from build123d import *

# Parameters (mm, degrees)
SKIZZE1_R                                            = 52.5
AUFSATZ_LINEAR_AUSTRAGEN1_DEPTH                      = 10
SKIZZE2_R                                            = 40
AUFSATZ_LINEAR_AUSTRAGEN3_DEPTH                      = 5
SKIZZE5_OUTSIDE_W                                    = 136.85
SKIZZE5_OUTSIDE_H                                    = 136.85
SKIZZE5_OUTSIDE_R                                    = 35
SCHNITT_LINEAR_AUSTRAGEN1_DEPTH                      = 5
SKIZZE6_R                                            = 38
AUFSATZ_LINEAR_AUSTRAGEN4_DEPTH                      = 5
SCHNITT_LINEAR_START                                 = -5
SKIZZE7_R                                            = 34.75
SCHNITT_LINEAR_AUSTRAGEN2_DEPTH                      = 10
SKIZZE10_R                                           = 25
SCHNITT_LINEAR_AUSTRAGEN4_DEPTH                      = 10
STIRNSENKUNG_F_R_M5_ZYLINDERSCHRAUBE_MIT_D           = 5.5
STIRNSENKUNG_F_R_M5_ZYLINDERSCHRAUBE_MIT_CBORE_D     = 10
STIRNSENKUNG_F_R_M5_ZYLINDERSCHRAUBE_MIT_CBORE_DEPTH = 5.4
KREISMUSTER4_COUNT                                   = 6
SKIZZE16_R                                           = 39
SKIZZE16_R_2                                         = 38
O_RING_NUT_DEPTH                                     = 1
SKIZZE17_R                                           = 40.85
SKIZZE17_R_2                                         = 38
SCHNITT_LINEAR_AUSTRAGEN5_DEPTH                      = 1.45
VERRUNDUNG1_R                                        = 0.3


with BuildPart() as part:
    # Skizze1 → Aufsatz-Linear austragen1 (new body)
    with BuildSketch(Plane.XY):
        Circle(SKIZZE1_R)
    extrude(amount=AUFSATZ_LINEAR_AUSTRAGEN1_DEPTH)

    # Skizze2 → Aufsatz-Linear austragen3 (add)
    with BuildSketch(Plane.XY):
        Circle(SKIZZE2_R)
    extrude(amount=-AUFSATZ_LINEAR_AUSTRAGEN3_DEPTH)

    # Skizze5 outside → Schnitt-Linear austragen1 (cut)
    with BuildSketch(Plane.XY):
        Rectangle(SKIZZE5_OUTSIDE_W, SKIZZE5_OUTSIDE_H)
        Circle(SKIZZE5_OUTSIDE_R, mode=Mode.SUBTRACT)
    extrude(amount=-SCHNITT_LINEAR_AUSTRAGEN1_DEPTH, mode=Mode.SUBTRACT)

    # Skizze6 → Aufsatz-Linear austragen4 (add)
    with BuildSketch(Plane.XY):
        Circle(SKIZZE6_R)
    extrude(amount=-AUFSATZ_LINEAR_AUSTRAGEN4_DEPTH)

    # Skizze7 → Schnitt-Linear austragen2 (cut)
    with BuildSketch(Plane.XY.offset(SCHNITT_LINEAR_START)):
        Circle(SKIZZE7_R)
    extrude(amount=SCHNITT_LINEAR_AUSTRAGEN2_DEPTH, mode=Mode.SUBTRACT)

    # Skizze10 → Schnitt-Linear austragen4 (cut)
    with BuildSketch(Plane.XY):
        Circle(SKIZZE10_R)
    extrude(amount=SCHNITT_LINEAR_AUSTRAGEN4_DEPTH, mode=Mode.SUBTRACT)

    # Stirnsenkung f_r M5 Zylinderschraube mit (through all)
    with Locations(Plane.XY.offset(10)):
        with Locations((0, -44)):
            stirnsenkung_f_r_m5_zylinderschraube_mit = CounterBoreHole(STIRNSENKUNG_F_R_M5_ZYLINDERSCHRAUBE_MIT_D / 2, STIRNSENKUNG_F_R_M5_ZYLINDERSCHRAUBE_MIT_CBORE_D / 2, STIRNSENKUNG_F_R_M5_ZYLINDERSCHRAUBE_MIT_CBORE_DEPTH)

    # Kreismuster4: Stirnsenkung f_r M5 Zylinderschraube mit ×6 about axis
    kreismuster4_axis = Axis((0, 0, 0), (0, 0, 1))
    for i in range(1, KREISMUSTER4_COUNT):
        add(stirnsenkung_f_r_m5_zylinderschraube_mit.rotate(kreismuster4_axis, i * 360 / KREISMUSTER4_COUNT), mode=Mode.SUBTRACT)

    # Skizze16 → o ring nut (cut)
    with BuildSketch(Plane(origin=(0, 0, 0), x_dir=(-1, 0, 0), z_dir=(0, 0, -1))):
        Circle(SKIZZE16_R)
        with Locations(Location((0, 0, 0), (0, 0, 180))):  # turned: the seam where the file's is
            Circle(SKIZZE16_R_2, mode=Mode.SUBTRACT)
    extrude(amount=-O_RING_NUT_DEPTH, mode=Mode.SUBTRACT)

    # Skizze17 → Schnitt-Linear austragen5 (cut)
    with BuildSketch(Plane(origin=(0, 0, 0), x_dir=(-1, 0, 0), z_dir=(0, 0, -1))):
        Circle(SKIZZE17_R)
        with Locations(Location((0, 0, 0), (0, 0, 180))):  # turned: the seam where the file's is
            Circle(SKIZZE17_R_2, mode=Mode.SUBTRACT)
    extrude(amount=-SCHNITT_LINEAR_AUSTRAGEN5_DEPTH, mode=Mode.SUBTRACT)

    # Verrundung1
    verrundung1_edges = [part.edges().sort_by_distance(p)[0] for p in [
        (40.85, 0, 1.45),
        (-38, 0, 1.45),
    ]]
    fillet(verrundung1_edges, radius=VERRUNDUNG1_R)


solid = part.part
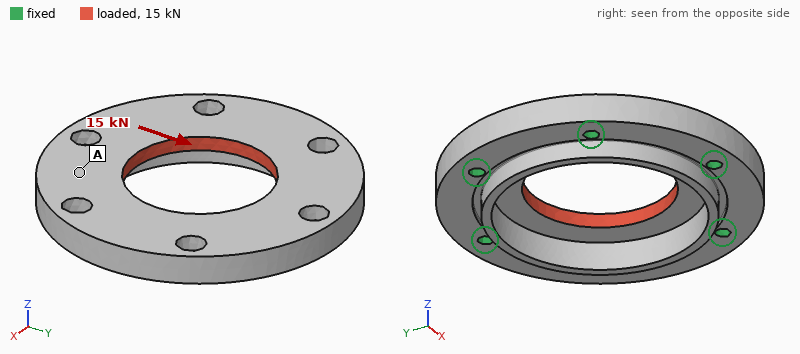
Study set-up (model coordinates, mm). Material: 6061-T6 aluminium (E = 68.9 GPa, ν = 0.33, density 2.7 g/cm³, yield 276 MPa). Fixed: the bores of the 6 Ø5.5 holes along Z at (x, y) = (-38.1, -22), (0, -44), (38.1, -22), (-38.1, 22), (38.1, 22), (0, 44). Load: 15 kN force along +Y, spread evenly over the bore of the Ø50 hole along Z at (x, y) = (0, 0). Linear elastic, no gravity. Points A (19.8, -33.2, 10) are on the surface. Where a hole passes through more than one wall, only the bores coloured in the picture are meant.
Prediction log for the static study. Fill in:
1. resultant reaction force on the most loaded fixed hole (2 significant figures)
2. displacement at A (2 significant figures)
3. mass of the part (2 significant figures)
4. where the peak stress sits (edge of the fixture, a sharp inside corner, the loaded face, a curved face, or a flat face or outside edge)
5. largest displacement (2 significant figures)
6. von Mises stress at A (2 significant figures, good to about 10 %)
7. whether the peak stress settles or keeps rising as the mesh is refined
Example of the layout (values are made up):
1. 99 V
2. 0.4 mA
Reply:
1. 2.7 kN
2. 14 µm
3. 150 g
4. edge of the fixture
5. 29 µm
6. 13 MPa
7. keeps rising
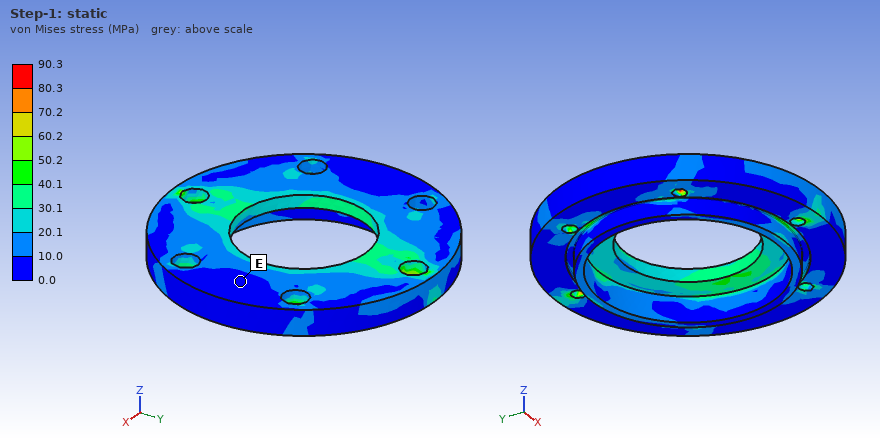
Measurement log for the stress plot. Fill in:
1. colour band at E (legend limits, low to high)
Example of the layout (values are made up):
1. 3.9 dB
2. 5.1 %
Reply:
1. 0.0 to 10.0 MPa
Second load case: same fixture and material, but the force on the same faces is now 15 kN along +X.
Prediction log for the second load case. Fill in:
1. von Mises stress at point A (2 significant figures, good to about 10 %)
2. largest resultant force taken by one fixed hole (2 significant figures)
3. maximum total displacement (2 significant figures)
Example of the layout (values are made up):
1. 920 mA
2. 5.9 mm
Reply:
1. 7.7 MPa
2. 2.6 kN
3. 29 µm
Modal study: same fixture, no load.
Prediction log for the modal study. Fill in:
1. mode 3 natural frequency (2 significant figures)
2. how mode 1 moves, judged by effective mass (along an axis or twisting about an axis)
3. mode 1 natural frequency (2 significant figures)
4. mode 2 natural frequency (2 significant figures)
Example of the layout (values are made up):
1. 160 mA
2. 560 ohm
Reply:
1. 14 kHz
2. along Z
3. 12 kHz
4. 13 kHz
